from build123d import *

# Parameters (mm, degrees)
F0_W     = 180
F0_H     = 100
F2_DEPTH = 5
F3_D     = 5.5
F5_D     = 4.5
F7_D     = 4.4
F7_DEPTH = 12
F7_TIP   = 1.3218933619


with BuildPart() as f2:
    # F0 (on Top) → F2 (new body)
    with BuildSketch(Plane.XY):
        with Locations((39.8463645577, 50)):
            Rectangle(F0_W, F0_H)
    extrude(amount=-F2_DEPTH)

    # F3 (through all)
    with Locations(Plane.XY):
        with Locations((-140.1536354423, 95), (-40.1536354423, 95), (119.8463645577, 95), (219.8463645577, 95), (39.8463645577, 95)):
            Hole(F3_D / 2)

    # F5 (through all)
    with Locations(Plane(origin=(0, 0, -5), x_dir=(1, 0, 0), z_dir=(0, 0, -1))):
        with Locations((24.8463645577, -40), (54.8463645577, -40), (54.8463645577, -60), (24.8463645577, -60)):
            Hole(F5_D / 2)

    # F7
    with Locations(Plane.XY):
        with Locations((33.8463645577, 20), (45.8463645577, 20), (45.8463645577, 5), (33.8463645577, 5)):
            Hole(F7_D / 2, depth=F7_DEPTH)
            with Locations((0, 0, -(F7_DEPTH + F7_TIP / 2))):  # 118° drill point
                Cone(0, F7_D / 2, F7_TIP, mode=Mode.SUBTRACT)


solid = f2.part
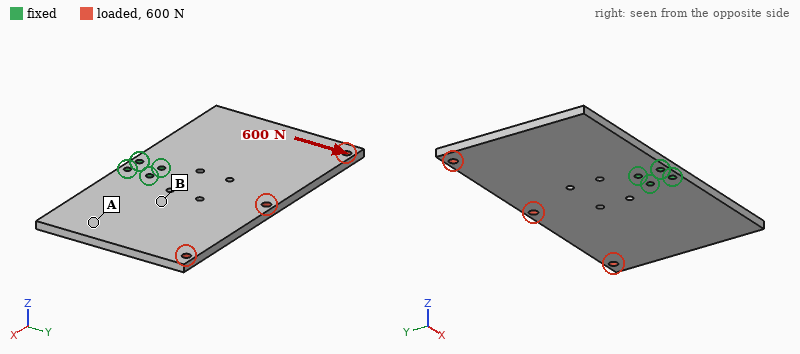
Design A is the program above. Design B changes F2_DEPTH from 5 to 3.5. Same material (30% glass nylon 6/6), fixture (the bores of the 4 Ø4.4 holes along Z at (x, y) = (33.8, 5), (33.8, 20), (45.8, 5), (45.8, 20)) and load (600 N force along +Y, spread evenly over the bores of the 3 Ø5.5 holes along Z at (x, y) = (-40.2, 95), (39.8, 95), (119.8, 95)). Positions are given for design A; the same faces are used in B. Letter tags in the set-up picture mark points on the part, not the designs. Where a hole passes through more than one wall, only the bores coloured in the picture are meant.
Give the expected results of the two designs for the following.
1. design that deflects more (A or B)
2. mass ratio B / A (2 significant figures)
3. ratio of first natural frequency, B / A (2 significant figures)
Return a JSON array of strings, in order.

["B", "0.70", "0.71"]
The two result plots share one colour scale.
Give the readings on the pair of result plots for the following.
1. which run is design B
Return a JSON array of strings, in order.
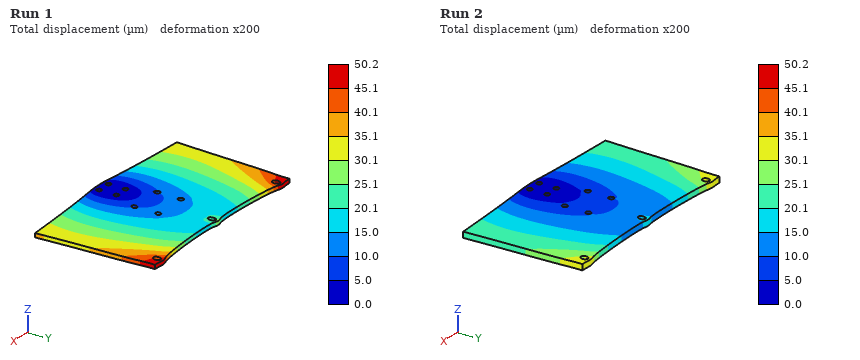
["Run 1"]
